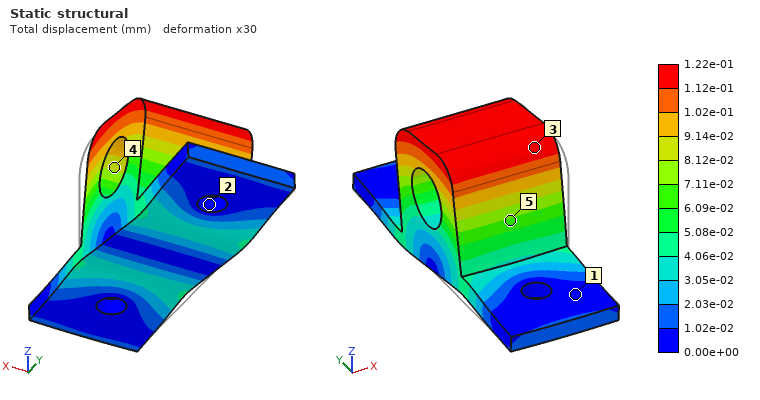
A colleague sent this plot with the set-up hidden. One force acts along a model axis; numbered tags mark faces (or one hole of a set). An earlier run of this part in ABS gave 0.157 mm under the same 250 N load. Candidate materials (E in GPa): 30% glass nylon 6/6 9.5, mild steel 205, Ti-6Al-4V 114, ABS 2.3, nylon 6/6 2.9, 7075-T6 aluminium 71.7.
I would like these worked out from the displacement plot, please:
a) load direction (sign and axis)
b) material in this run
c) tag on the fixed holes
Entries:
+Y
nylon 6/6
2
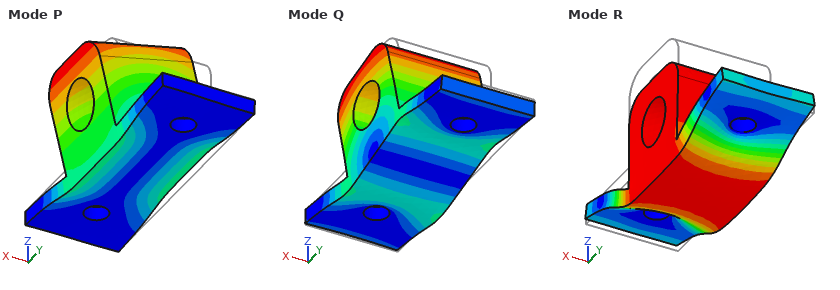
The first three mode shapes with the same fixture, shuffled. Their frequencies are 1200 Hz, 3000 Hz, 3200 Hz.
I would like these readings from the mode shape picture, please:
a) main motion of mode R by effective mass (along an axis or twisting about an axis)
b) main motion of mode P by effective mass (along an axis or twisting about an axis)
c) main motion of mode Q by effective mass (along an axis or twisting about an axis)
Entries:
along Z
along X
along Y
